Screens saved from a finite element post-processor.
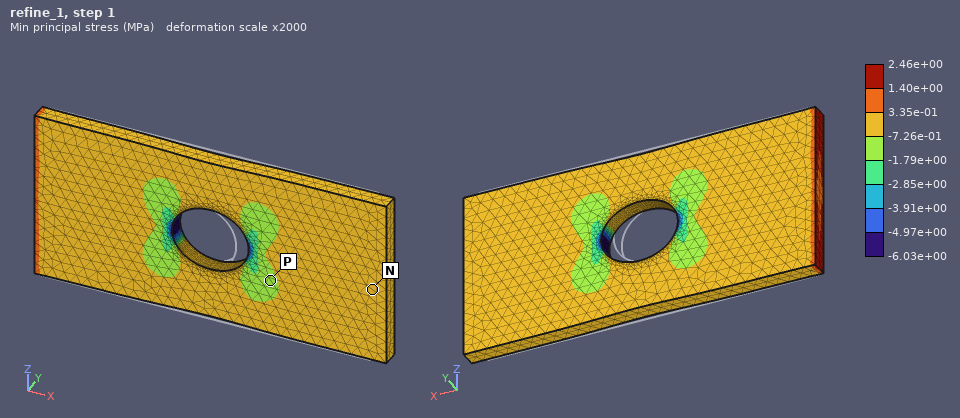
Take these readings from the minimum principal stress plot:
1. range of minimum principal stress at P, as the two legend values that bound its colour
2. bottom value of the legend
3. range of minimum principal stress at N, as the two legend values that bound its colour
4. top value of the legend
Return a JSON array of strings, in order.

["-1.79e+00 to -7.26e-01 MPa", "-6.03e+00 MPa", "-7.26e-01 to 3.35e-01 MPa", "2.46e+00 MPa"]
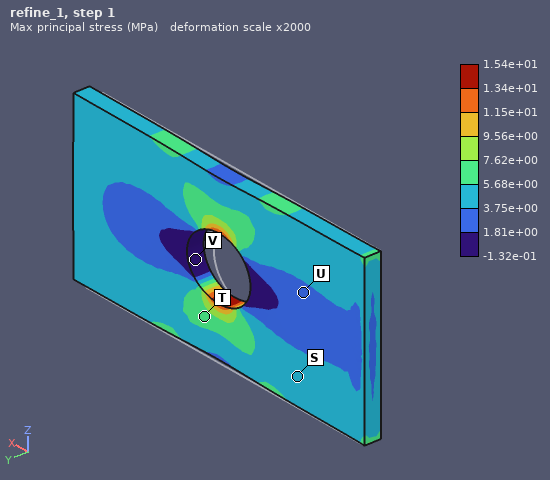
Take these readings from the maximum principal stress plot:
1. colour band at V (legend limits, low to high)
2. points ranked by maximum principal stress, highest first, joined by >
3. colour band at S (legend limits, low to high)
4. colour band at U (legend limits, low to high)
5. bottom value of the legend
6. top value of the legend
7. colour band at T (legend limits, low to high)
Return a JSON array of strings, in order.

["-1.32e-01 to 1.81e+00 MPa", "T > S > U > V", "3.75e+00 to 5.68e+00 MPa", "1.81e+00 to 3.75e+00 MPa", "-1.32e-01 MPa", "1.54e+01 MPa", "5.68e+00 to 7.62e+00 MPa"]
